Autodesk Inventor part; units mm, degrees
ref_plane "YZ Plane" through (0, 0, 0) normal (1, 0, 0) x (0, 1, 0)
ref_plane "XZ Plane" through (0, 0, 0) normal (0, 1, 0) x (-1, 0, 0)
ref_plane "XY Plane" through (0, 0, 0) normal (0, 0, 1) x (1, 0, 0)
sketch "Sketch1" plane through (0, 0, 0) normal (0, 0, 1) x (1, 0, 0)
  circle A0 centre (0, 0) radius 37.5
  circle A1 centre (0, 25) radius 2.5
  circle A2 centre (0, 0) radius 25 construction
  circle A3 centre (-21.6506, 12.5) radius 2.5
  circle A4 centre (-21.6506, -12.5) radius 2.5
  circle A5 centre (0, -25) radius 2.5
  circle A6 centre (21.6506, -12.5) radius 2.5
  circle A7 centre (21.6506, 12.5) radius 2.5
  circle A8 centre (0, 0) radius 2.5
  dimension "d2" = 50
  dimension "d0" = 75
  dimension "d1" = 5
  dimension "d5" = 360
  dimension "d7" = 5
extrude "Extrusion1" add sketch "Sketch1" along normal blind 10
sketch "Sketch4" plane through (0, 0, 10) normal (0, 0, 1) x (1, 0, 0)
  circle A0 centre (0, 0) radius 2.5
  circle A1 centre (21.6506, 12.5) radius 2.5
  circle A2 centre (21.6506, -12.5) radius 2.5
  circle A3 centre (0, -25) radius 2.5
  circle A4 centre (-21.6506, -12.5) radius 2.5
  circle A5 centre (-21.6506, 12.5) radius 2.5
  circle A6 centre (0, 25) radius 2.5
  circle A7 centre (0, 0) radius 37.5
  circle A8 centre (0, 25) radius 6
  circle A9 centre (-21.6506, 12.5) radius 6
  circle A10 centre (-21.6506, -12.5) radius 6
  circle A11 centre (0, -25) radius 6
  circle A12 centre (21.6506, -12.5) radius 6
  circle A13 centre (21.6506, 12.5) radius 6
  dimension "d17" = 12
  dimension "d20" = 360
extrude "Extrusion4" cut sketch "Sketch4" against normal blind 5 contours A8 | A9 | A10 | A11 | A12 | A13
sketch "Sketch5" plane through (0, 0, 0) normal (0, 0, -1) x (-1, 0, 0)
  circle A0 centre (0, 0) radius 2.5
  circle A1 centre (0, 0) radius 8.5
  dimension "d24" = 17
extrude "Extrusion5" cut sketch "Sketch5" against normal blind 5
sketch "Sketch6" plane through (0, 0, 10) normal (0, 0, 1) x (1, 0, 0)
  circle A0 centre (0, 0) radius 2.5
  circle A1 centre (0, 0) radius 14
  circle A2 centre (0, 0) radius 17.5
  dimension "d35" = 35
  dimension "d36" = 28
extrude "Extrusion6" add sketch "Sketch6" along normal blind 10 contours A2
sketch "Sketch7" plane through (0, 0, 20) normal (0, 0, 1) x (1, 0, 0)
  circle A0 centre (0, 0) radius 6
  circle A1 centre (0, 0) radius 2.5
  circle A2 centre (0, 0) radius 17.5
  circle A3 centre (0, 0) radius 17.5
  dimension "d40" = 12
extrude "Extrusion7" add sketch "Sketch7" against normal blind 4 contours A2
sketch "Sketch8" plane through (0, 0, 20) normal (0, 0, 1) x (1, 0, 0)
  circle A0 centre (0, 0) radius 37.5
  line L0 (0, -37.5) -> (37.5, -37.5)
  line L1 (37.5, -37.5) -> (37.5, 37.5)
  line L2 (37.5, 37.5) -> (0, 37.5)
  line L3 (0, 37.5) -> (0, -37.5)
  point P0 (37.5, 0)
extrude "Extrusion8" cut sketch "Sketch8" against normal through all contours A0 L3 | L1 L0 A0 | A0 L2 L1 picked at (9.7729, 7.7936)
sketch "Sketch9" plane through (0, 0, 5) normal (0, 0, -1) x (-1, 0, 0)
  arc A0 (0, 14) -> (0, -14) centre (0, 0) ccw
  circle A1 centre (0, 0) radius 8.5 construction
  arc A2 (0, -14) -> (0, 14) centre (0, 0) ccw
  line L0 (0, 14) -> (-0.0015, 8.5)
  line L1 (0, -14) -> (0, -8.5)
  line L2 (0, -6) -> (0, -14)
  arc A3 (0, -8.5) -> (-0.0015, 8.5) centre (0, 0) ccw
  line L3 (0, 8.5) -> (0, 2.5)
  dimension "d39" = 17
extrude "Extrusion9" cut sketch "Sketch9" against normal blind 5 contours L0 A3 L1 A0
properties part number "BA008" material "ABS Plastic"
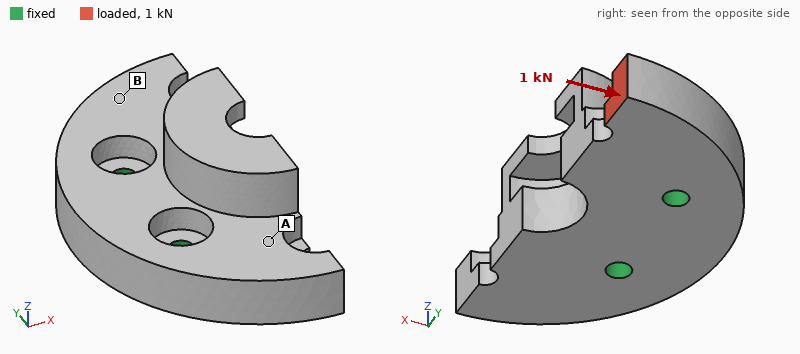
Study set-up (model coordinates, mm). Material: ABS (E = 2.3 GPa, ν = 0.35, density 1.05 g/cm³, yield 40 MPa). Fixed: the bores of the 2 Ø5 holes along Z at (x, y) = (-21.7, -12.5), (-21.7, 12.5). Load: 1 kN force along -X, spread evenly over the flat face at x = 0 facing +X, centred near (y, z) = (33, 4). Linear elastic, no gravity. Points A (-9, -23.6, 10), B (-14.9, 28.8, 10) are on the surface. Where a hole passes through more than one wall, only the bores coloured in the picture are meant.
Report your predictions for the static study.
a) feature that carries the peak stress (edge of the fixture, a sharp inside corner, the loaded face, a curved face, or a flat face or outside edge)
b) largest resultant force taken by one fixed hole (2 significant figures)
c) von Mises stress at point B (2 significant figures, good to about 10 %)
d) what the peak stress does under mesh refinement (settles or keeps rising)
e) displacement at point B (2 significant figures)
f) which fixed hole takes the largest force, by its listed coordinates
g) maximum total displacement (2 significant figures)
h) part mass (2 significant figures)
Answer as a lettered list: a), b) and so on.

a) edge of the fixture
b) 1.7 kN
c) 9.3 MPa
d) keeps rising
e) 0.37 mm
f) (-21.7, 12.5)
g) 0.76 mm
h) 23 g
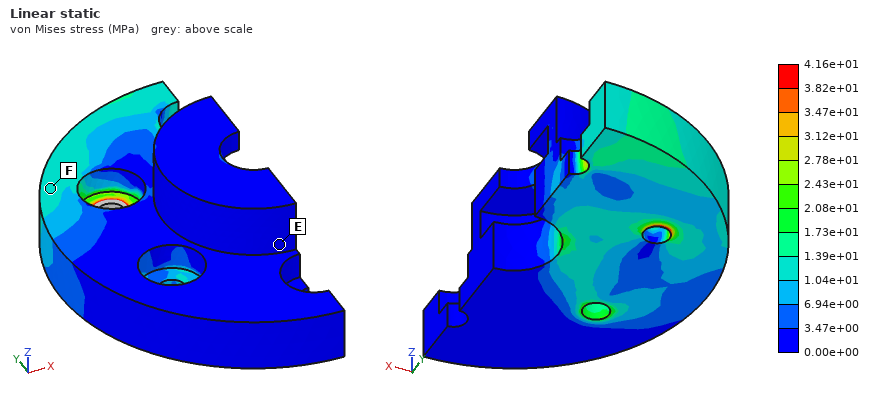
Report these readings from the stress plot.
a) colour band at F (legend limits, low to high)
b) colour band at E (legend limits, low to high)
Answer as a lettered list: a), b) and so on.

a) 1.04e+01 to 1.39e+01 MPa
b) 0.00e+00 to 3.47e+00 MPa
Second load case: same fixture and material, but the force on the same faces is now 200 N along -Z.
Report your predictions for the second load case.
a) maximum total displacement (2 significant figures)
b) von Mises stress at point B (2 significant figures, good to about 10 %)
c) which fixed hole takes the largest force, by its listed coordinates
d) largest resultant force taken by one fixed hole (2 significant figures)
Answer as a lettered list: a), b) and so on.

a) 0.87 mm
b) 8.9 MPa
c) (-21.7, 12.5)
d) 340 N
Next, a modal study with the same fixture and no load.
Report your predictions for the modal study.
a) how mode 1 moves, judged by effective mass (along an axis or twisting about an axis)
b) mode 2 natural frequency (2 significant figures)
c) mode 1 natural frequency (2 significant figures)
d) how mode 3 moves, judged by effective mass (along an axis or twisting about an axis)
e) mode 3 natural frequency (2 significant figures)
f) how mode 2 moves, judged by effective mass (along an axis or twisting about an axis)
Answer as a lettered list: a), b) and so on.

a) along Z
b) 2300 Hz
c) 1700 Hz
d) along Y
e) 3400 Hz
f) twisting about X
